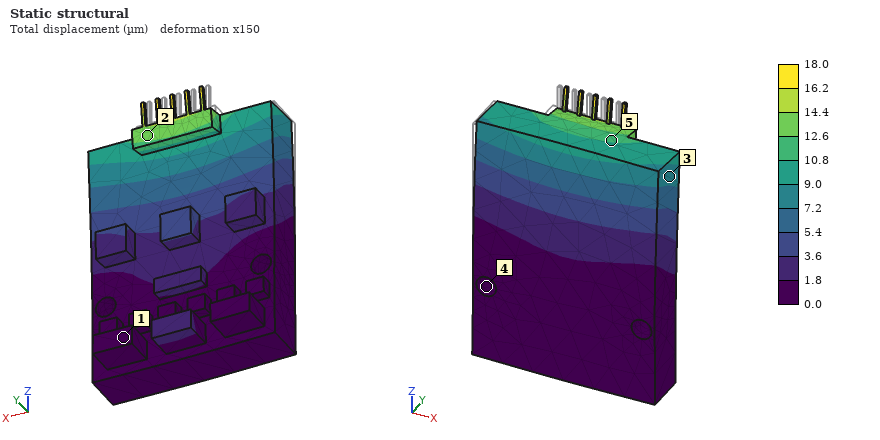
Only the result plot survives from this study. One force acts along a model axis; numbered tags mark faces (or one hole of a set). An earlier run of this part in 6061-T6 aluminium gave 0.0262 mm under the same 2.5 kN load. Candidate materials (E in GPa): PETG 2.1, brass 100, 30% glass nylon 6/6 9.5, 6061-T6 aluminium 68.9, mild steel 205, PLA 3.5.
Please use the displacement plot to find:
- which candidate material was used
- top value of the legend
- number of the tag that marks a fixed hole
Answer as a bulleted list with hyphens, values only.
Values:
- brass
- 18.0 µm
- 4
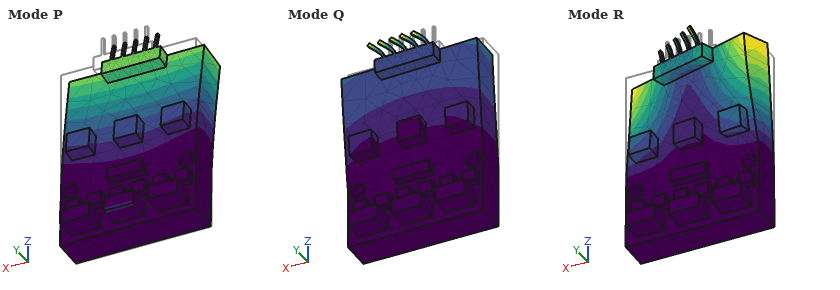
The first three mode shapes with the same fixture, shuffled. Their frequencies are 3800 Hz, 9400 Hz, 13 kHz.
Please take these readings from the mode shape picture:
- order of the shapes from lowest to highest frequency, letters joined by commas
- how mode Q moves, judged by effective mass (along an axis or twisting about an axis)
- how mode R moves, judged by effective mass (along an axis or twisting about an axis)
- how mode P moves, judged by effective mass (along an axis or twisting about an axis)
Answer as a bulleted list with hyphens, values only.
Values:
- P, R, Q
- along X
- twisting about Z
- along Y
